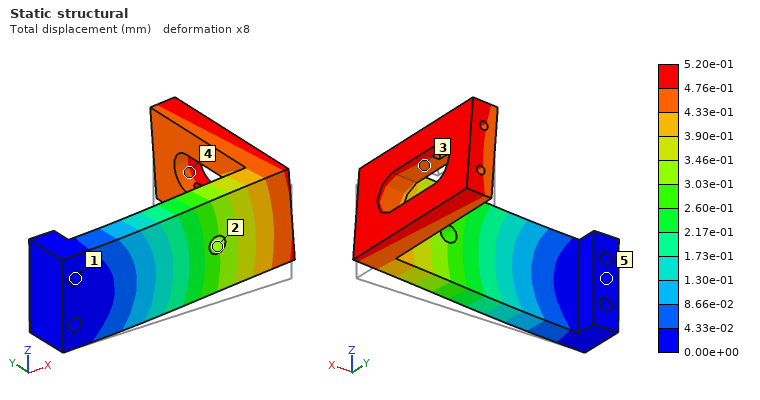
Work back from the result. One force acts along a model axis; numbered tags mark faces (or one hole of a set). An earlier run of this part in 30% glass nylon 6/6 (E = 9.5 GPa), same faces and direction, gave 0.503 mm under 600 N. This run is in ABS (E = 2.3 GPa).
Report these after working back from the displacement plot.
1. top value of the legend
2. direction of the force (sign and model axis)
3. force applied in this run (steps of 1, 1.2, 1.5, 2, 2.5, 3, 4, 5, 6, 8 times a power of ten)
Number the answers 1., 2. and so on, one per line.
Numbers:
1. 5.20e-01 mm
2. +Z
3. 150 N
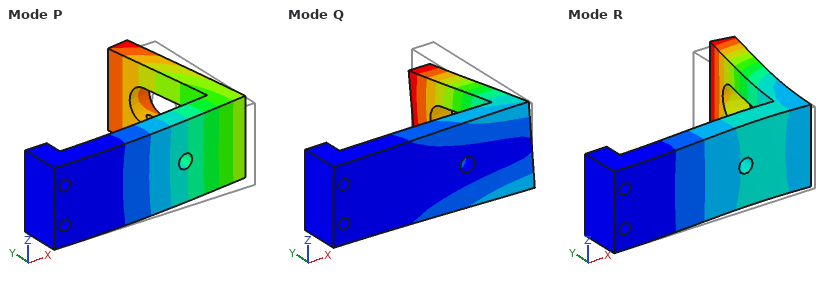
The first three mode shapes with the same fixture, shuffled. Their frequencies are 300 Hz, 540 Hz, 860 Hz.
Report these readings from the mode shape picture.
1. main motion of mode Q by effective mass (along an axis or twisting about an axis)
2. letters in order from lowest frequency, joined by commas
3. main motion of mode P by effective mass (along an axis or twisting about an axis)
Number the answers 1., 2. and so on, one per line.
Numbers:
1. along Z
2. P, Q, R
3. along Y
